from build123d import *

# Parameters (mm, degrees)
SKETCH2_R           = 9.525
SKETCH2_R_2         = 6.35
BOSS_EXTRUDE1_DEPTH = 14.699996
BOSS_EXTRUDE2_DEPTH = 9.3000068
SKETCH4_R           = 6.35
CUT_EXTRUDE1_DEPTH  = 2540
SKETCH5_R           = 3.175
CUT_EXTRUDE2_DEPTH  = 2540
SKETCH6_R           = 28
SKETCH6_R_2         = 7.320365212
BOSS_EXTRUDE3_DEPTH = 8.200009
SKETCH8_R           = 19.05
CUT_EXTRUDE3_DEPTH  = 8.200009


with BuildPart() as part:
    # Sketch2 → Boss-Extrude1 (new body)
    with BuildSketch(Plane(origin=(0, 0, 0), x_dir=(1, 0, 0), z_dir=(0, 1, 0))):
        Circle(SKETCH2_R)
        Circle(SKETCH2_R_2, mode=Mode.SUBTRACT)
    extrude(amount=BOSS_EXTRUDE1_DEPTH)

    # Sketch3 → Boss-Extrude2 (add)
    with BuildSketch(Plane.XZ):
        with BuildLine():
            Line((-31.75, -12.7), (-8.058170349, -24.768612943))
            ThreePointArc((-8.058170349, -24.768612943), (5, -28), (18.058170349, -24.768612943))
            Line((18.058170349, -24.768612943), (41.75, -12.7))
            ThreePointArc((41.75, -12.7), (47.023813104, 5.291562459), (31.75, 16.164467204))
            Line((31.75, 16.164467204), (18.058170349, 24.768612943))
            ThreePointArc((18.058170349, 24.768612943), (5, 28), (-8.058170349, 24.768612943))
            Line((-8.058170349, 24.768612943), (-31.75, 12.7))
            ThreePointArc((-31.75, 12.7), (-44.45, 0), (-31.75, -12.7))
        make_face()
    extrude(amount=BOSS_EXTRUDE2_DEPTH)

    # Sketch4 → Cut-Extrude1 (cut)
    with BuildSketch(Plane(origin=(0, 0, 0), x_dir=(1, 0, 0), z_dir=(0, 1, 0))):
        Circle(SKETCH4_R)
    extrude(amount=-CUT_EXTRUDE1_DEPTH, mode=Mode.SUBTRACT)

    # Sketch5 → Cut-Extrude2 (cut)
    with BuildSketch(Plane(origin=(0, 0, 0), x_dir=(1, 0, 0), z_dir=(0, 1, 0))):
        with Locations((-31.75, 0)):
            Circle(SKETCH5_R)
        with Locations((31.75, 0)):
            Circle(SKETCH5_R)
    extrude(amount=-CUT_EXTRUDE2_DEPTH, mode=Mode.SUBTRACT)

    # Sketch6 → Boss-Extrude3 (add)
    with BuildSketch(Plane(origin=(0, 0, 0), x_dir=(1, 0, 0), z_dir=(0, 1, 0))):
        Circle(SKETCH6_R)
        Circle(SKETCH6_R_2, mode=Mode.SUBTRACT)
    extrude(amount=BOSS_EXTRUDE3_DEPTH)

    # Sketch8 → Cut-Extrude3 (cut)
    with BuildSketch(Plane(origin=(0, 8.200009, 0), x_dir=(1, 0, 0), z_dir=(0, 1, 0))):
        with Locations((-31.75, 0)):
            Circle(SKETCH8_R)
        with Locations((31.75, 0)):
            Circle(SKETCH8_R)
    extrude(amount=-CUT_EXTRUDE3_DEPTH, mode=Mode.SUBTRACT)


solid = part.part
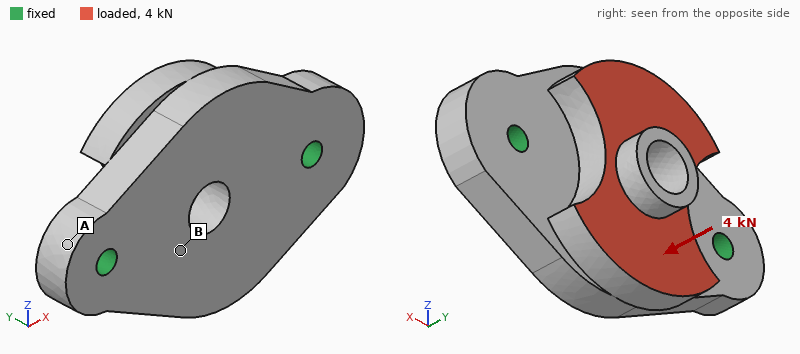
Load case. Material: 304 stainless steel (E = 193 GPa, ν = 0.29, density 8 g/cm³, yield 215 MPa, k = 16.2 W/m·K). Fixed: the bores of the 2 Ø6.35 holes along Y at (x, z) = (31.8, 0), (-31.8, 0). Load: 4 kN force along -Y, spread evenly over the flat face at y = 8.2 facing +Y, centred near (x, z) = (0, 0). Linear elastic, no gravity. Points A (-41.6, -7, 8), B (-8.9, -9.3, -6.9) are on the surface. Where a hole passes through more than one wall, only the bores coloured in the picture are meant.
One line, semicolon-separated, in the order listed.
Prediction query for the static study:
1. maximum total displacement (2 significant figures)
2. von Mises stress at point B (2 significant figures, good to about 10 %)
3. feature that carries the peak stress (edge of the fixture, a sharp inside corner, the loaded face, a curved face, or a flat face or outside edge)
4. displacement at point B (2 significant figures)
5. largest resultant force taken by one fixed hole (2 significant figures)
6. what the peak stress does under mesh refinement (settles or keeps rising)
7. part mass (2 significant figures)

8.7 µm; 18 MPa; edge of the fixture; 6.1 µm; 2.2 kN; keeps rising; 360 g
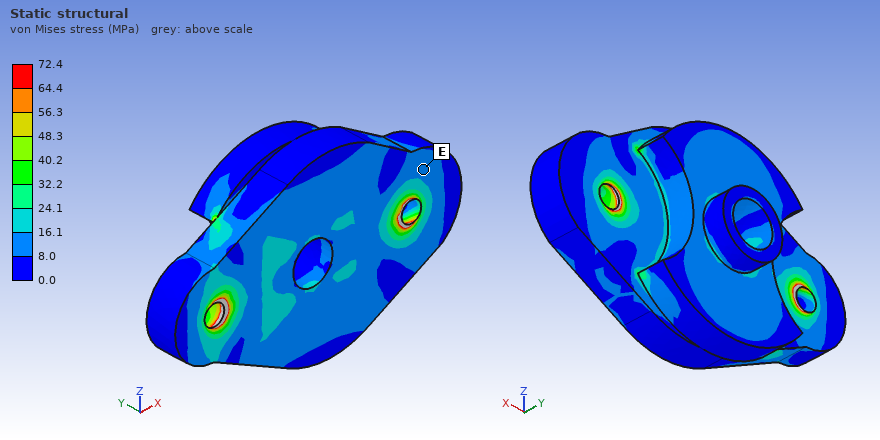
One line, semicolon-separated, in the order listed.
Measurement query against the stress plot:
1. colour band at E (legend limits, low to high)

8.0 to 16.1 MPa
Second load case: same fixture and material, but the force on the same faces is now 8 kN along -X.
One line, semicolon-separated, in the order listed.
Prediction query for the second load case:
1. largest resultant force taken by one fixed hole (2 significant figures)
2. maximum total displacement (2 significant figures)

4.6 kN; 7.4 µm
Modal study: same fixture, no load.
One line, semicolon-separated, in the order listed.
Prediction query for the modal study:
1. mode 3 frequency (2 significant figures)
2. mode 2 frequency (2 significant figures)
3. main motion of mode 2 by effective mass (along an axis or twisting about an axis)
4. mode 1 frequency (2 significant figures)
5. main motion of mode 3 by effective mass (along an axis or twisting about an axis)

14 kHz; 7600 Hz; along Y; 5100 Hz; along Z
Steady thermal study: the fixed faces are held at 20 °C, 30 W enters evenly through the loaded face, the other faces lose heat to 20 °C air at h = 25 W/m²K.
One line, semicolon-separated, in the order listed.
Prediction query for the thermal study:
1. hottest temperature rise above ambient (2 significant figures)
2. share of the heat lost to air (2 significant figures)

61 K; 29 %
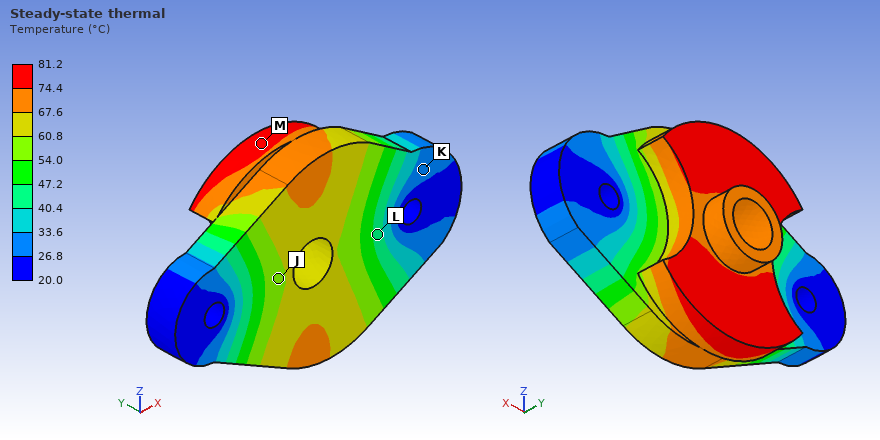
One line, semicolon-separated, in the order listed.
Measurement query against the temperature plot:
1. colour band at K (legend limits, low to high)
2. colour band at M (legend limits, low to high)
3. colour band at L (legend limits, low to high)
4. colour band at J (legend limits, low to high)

26.8 to 33.6 °C; 74.4 to 81.2 °C; 40.4 to 47.2 °C; 54.0 to 60.8 °C
